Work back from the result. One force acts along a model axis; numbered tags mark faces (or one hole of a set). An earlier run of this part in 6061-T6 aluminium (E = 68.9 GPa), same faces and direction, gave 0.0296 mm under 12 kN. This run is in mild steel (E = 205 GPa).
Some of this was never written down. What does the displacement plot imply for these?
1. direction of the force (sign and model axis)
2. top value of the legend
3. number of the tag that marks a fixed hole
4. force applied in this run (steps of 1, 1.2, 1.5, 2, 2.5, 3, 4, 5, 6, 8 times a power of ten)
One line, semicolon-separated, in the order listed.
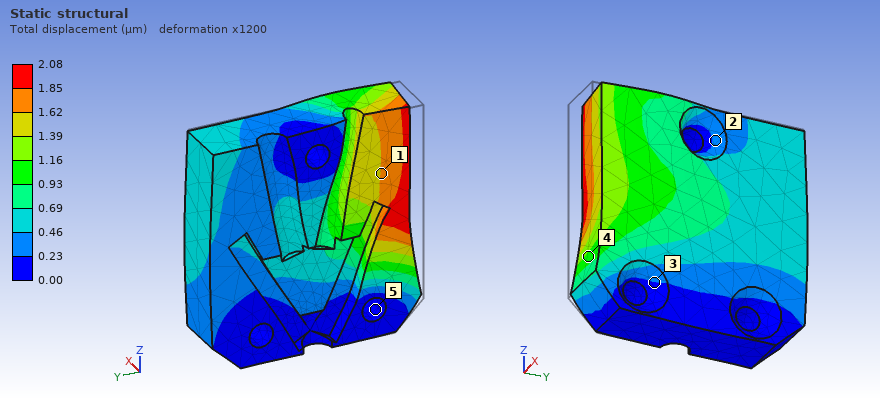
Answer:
+Y; 2.08 µm; 5; 2.5 kN
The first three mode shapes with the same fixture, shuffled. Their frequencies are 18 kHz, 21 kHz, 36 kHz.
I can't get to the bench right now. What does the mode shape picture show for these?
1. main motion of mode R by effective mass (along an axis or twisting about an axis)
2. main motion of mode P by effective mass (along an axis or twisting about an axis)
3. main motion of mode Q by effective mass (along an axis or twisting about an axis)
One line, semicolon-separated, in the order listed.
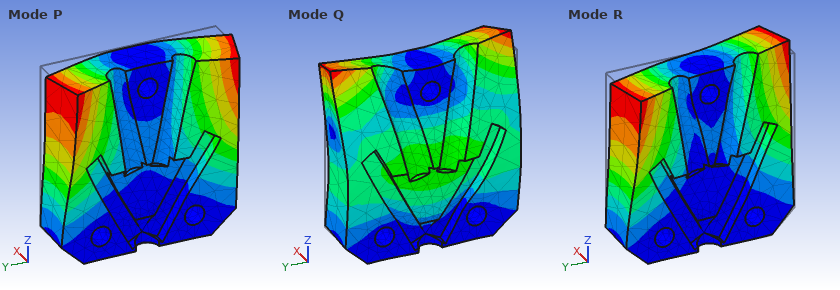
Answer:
twisting about Z; along X; along X
